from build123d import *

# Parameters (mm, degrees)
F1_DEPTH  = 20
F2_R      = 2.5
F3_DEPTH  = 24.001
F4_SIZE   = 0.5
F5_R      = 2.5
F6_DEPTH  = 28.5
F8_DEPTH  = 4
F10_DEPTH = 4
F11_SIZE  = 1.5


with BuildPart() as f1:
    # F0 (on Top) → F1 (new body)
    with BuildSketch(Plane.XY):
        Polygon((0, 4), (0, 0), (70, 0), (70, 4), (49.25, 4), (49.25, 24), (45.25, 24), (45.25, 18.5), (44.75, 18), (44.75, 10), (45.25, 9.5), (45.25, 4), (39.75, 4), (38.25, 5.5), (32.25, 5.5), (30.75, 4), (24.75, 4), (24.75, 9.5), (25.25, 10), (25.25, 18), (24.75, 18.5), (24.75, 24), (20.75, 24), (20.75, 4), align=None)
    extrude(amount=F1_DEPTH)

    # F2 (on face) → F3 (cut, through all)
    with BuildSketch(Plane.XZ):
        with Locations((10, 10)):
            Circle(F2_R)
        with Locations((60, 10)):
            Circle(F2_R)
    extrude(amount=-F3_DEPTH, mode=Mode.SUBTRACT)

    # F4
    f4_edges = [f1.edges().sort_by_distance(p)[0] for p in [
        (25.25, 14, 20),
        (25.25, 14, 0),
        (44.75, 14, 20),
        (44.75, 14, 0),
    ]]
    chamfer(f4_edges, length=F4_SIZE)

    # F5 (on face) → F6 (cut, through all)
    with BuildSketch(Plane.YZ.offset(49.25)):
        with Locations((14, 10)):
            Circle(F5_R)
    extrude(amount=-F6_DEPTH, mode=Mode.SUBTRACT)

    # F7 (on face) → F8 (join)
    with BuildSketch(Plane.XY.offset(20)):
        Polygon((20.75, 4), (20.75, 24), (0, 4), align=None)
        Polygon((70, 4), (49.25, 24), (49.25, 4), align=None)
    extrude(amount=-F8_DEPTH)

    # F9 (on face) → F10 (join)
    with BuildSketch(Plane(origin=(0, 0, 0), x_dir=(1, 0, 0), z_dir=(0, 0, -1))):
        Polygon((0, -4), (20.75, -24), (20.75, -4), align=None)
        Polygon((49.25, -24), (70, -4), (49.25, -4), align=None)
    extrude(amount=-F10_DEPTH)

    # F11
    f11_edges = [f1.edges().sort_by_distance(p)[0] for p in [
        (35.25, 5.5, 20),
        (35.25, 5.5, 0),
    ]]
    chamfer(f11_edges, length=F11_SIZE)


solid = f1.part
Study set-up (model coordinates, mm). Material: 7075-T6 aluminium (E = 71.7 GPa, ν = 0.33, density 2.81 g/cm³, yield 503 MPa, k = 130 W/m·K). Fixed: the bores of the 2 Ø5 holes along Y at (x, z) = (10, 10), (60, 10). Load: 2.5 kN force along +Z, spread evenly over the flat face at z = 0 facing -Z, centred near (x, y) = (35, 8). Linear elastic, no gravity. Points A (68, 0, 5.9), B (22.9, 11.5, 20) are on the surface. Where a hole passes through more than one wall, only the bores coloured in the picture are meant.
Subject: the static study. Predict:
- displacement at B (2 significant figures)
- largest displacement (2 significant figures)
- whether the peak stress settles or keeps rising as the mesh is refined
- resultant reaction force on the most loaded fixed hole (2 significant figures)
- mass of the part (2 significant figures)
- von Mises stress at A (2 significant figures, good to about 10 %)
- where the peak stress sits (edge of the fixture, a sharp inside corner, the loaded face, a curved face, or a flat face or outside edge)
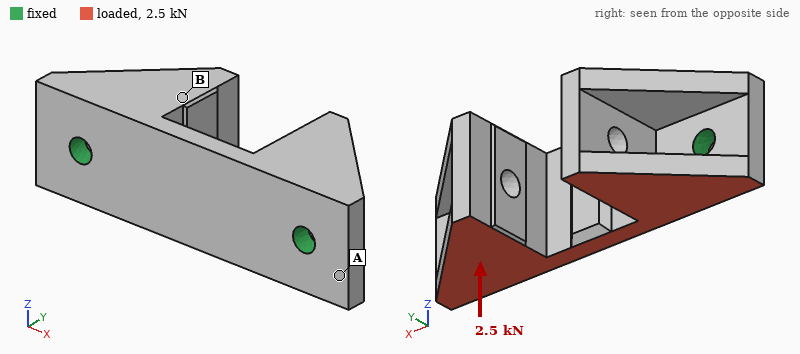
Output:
46 µm
84 µm
keeps rising
1.3 kN
34 g
37 MPa
edge of the fixture
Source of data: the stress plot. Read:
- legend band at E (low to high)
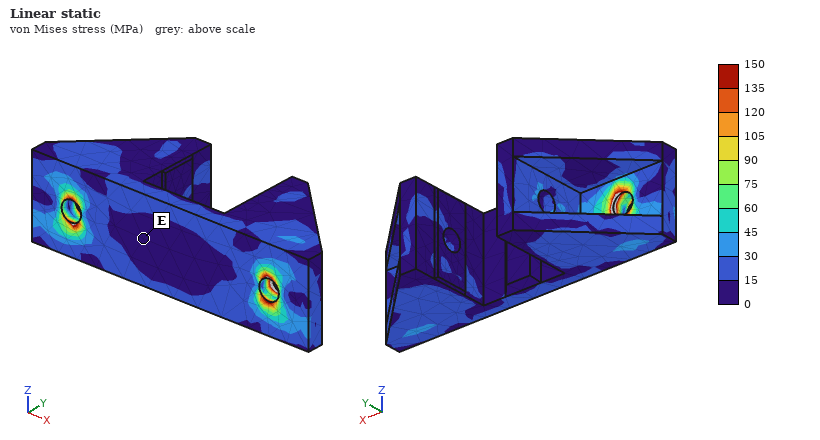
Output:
0 to 15 MPa
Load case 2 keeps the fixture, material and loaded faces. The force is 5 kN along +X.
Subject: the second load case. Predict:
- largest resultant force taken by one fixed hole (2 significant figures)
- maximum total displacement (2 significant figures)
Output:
2.7 kN
70 µm
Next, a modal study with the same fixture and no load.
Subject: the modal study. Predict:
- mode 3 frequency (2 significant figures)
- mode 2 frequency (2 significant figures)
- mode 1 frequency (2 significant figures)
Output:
7900 Hz
6000 Hz
5900 Hz
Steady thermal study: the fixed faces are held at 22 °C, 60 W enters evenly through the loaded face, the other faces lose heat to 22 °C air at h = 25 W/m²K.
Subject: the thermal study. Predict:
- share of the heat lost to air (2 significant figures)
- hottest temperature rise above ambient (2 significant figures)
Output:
3.9 %
28 K
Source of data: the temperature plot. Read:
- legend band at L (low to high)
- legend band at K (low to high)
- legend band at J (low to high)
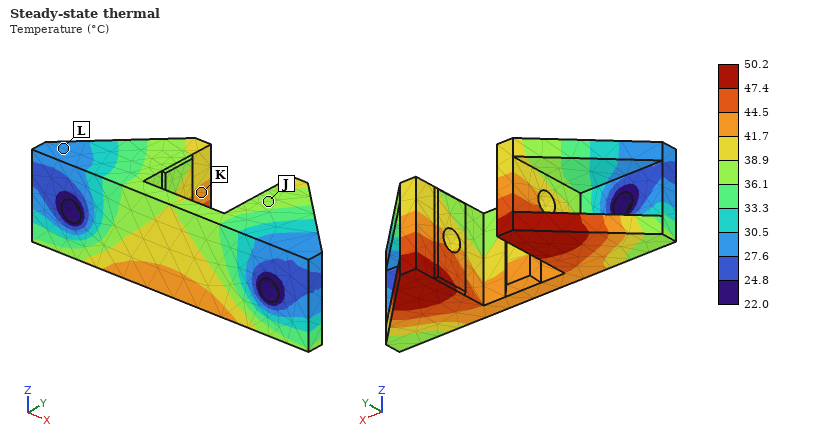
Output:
27.6 to 30.5 °C
41.7 to 44.5 °C
36.1 to 38.9 °C
